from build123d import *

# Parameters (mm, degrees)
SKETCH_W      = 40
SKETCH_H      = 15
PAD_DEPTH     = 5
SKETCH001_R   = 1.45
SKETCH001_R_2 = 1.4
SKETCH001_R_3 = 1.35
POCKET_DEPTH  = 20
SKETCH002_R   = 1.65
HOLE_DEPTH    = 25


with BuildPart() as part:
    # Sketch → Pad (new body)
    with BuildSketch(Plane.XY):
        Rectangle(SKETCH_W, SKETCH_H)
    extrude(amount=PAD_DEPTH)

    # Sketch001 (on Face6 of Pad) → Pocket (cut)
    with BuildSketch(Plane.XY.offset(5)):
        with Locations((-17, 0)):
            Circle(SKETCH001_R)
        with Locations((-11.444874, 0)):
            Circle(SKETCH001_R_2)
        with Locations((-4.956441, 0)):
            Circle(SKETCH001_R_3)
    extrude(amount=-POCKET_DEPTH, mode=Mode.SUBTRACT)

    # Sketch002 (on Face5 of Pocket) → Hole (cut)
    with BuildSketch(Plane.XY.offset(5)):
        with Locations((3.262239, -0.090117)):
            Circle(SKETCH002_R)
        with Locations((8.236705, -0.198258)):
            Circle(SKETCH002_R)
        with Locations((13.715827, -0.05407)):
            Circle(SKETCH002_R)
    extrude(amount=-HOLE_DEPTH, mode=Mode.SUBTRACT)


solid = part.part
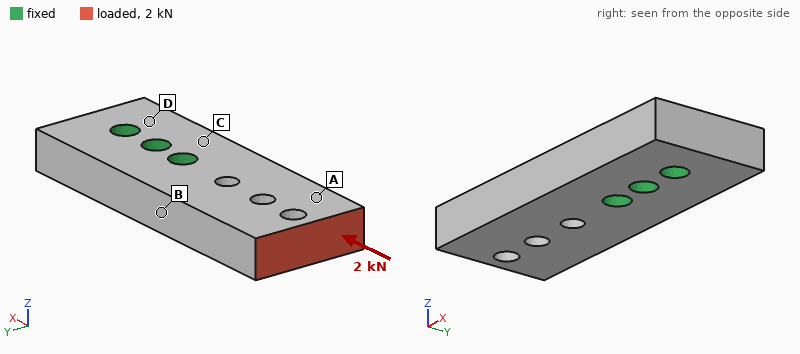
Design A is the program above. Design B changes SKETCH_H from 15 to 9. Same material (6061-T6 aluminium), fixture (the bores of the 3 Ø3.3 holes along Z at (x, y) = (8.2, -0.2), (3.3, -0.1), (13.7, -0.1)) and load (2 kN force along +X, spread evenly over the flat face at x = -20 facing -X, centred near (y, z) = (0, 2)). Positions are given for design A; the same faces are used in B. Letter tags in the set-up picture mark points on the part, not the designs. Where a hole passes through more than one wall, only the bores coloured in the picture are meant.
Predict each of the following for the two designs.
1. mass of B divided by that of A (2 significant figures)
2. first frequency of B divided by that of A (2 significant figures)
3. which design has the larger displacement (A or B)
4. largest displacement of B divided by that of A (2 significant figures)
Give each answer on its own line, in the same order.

0.57
1.1
B
1.7
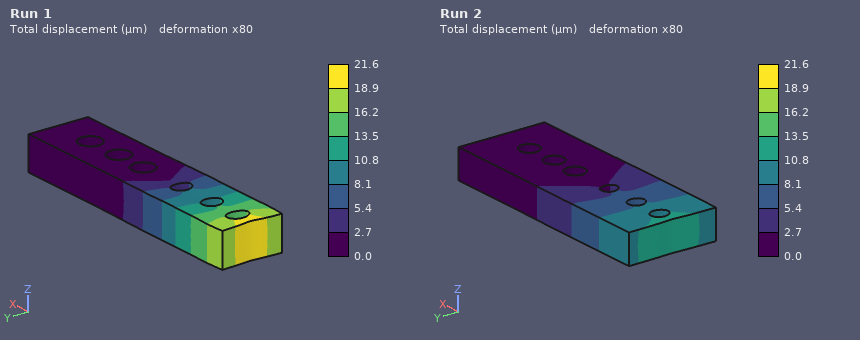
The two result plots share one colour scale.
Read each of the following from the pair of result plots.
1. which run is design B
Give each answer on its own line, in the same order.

Run 1
